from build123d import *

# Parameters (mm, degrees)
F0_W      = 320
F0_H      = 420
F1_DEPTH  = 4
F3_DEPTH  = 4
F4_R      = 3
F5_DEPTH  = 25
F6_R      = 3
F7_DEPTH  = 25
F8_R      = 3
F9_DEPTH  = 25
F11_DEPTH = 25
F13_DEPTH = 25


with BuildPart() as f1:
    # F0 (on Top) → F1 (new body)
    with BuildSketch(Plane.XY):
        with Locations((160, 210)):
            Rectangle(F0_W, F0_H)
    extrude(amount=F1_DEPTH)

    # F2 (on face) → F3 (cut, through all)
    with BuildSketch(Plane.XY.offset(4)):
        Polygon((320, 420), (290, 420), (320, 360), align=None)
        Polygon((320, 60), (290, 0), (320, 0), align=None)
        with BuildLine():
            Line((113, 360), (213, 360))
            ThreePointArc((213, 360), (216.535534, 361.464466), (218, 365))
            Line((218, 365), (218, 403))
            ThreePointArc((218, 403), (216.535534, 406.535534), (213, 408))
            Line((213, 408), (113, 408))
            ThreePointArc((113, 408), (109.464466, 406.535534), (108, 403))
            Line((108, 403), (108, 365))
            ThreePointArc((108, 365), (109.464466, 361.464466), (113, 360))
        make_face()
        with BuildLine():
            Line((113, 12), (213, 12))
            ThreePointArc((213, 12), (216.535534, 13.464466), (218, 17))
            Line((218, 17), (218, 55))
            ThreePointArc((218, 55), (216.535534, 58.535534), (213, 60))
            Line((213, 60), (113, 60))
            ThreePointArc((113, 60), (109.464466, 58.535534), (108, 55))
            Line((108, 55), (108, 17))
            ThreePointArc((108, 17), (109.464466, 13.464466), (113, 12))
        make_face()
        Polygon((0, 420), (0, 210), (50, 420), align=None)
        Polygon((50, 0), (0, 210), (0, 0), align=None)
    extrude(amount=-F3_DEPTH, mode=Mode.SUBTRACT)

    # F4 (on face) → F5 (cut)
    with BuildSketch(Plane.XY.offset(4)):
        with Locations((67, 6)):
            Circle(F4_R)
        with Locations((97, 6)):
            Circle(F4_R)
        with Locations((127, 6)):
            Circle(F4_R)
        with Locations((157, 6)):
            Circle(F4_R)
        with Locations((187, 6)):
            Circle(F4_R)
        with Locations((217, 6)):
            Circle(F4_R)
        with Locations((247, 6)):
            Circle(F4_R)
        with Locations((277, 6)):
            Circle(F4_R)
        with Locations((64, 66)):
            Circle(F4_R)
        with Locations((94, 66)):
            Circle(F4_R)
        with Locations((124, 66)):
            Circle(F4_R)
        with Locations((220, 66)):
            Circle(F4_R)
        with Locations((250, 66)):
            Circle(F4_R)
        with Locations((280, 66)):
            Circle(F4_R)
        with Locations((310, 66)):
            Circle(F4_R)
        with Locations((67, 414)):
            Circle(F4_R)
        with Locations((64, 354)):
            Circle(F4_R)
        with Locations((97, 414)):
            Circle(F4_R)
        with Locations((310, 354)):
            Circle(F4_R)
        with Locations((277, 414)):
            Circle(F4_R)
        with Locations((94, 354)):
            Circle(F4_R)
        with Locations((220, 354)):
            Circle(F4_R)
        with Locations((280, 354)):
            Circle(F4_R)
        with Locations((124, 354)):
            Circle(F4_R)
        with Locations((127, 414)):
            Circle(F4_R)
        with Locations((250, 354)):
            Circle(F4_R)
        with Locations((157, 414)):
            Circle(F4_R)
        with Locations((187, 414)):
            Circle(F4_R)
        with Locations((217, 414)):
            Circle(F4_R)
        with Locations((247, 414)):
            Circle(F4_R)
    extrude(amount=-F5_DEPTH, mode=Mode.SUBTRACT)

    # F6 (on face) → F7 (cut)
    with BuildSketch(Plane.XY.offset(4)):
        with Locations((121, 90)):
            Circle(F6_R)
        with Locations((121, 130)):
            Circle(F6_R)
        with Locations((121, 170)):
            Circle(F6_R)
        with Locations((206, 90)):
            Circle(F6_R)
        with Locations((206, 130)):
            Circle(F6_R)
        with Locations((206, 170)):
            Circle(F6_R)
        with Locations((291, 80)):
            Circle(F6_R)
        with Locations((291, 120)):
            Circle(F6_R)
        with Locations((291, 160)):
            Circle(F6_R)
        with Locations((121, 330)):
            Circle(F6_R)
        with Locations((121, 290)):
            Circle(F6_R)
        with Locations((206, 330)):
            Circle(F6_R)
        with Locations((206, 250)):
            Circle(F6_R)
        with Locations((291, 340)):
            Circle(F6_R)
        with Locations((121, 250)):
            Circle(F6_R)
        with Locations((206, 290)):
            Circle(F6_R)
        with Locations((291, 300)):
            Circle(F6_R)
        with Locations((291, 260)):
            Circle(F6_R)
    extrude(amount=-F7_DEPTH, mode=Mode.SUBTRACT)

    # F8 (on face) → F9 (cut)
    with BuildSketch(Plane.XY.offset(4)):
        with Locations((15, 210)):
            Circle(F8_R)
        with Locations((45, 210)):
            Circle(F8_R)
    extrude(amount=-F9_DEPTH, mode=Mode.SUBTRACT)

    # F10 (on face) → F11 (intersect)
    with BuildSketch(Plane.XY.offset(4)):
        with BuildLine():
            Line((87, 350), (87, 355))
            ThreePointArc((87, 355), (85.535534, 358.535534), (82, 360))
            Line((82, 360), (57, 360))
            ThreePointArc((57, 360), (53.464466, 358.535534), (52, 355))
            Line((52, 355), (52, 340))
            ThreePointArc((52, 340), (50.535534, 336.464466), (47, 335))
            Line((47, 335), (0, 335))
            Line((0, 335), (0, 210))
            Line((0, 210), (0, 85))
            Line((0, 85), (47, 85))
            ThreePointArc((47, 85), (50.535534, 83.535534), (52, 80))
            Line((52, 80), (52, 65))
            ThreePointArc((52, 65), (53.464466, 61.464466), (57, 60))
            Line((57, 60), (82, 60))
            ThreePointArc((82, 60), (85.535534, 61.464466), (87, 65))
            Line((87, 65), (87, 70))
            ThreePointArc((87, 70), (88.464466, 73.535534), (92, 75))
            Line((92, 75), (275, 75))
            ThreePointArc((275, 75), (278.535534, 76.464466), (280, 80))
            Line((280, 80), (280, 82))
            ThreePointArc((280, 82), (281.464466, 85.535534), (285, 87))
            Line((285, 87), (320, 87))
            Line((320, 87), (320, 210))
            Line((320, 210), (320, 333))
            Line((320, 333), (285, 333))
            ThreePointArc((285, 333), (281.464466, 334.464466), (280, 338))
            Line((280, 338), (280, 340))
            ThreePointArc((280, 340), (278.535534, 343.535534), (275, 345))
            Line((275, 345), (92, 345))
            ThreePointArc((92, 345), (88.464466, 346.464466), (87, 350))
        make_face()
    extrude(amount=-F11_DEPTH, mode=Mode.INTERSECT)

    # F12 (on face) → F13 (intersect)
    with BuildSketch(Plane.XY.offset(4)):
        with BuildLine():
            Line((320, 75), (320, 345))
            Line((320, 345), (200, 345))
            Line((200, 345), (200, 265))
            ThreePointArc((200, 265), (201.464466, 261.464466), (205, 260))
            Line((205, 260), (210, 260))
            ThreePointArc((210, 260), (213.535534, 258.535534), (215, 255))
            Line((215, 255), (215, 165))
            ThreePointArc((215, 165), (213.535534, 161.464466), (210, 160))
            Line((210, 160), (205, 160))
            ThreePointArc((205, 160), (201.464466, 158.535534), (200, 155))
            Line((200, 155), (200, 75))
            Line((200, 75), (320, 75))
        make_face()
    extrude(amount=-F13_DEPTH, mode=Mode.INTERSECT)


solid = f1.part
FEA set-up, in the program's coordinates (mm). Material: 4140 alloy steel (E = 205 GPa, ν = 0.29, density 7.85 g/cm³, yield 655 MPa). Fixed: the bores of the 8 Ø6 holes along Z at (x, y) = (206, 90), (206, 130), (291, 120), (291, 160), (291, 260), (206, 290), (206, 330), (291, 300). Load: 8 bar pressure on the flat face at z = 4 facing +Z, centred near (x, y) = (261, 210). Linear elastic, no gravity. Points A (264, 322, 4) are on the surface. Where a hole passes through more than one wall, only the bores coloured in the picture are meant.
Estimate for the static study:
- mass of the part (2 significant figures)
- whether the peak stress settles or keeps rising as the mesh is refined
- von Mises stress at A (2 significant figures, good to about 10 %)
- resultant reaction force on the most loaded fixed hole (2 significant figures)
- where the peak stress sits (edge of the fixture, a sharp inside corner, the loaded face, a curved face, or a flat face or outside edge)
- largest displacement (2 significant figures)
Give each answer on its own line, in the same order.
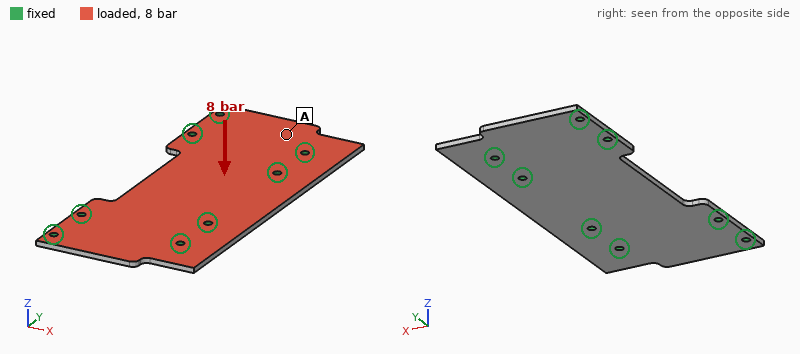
930 g
keeps rising
91 MPa
4.7 kN
edge of the fixture
0.97 mm
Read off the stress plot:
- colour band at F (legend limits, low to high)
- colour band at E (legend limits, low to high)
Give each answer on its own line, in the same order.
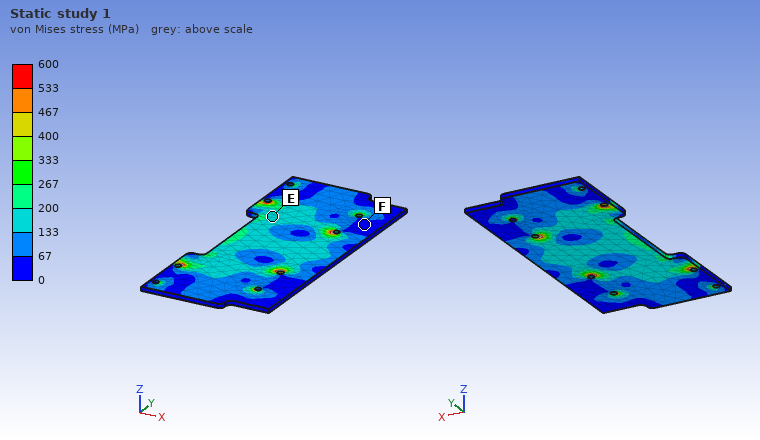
0 to 67 MPa
133 to 200 MPa
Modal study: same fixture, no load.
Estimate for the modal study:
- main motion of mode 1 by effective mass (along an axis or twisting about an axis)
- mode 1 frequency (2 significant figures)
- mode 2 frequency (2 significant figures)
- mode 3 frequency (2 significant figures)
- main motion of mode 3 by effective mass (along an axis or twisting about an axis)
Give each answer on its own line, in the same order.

along Z
1100 Hz
1900 Hz
2000 Hz
along Z
